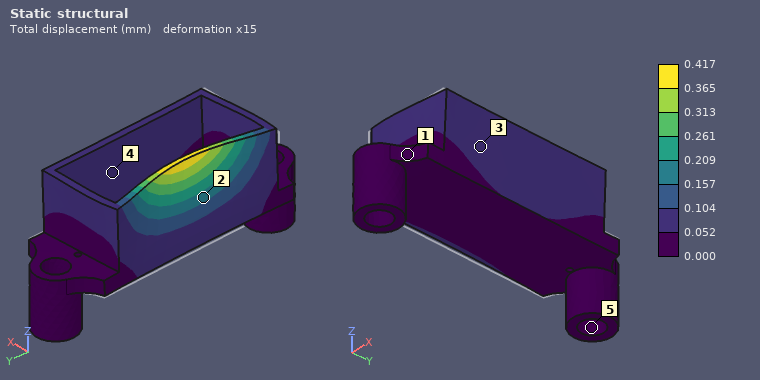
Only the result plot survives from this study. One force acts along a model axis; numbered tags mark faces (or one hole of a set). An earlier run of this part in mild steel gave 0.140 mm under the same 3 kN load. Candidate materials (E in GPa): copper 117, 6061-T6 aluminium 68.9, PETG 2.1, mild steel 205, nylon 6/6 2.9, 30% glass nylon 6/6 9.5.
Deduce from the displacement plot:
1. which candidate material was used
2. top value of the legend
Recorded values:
6061-T6 aluminium
0.417 mm
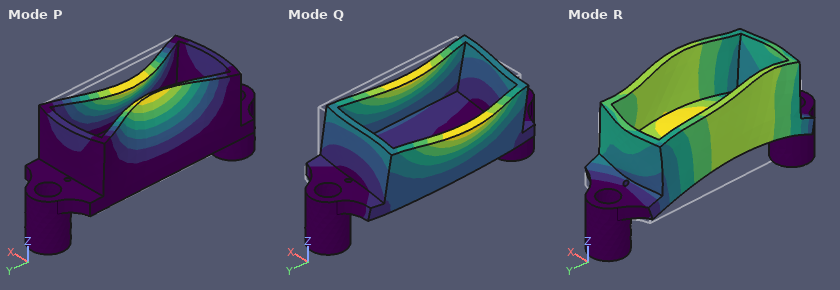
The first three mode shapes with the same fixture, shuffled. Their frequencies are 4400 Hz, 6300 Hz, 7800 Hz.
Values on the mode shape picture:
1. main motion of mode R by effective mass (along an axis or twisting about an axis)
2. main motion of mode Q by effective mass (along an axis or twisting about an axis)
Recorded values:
along Z
along X
